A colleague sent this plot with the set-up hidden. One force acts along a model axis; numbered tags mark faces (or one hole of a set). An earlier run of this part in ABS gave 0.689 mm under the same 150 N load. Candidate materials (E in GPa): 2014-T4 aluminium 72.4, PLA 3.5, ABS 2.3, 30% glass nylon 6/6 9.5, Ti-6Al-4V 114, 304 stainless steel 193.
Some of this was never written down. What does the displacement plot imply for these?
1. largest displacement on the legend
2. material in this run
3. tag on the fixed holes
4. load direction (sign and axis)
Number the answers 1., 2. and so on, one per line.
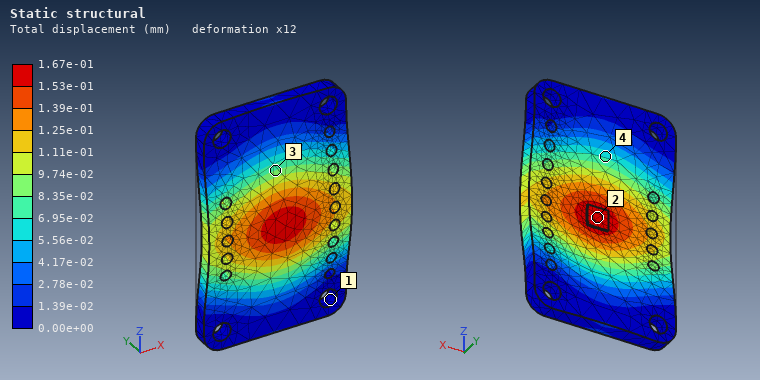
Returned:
1. 1.67e-01 mm
2. 30% glass nylon 6/6
3. 1
4. -Y
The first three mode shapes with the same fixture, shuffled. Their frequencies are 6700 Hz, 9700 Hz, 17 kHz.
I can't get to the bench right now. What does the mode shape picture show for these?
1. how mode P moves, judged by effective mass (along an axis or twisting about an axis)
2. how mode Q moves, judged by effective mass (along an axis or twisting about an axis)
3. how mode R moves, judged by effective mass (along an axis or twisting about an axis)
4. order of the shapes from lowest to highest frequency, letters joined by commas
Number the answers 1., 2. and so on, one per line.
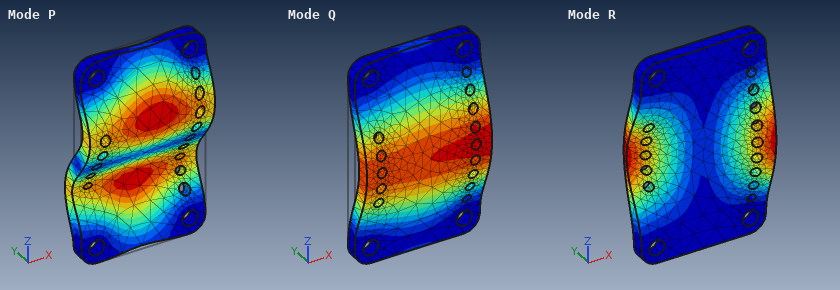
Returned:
1. twisting about X
2. along Y
3. twisting about Z
4. Q, R, P
